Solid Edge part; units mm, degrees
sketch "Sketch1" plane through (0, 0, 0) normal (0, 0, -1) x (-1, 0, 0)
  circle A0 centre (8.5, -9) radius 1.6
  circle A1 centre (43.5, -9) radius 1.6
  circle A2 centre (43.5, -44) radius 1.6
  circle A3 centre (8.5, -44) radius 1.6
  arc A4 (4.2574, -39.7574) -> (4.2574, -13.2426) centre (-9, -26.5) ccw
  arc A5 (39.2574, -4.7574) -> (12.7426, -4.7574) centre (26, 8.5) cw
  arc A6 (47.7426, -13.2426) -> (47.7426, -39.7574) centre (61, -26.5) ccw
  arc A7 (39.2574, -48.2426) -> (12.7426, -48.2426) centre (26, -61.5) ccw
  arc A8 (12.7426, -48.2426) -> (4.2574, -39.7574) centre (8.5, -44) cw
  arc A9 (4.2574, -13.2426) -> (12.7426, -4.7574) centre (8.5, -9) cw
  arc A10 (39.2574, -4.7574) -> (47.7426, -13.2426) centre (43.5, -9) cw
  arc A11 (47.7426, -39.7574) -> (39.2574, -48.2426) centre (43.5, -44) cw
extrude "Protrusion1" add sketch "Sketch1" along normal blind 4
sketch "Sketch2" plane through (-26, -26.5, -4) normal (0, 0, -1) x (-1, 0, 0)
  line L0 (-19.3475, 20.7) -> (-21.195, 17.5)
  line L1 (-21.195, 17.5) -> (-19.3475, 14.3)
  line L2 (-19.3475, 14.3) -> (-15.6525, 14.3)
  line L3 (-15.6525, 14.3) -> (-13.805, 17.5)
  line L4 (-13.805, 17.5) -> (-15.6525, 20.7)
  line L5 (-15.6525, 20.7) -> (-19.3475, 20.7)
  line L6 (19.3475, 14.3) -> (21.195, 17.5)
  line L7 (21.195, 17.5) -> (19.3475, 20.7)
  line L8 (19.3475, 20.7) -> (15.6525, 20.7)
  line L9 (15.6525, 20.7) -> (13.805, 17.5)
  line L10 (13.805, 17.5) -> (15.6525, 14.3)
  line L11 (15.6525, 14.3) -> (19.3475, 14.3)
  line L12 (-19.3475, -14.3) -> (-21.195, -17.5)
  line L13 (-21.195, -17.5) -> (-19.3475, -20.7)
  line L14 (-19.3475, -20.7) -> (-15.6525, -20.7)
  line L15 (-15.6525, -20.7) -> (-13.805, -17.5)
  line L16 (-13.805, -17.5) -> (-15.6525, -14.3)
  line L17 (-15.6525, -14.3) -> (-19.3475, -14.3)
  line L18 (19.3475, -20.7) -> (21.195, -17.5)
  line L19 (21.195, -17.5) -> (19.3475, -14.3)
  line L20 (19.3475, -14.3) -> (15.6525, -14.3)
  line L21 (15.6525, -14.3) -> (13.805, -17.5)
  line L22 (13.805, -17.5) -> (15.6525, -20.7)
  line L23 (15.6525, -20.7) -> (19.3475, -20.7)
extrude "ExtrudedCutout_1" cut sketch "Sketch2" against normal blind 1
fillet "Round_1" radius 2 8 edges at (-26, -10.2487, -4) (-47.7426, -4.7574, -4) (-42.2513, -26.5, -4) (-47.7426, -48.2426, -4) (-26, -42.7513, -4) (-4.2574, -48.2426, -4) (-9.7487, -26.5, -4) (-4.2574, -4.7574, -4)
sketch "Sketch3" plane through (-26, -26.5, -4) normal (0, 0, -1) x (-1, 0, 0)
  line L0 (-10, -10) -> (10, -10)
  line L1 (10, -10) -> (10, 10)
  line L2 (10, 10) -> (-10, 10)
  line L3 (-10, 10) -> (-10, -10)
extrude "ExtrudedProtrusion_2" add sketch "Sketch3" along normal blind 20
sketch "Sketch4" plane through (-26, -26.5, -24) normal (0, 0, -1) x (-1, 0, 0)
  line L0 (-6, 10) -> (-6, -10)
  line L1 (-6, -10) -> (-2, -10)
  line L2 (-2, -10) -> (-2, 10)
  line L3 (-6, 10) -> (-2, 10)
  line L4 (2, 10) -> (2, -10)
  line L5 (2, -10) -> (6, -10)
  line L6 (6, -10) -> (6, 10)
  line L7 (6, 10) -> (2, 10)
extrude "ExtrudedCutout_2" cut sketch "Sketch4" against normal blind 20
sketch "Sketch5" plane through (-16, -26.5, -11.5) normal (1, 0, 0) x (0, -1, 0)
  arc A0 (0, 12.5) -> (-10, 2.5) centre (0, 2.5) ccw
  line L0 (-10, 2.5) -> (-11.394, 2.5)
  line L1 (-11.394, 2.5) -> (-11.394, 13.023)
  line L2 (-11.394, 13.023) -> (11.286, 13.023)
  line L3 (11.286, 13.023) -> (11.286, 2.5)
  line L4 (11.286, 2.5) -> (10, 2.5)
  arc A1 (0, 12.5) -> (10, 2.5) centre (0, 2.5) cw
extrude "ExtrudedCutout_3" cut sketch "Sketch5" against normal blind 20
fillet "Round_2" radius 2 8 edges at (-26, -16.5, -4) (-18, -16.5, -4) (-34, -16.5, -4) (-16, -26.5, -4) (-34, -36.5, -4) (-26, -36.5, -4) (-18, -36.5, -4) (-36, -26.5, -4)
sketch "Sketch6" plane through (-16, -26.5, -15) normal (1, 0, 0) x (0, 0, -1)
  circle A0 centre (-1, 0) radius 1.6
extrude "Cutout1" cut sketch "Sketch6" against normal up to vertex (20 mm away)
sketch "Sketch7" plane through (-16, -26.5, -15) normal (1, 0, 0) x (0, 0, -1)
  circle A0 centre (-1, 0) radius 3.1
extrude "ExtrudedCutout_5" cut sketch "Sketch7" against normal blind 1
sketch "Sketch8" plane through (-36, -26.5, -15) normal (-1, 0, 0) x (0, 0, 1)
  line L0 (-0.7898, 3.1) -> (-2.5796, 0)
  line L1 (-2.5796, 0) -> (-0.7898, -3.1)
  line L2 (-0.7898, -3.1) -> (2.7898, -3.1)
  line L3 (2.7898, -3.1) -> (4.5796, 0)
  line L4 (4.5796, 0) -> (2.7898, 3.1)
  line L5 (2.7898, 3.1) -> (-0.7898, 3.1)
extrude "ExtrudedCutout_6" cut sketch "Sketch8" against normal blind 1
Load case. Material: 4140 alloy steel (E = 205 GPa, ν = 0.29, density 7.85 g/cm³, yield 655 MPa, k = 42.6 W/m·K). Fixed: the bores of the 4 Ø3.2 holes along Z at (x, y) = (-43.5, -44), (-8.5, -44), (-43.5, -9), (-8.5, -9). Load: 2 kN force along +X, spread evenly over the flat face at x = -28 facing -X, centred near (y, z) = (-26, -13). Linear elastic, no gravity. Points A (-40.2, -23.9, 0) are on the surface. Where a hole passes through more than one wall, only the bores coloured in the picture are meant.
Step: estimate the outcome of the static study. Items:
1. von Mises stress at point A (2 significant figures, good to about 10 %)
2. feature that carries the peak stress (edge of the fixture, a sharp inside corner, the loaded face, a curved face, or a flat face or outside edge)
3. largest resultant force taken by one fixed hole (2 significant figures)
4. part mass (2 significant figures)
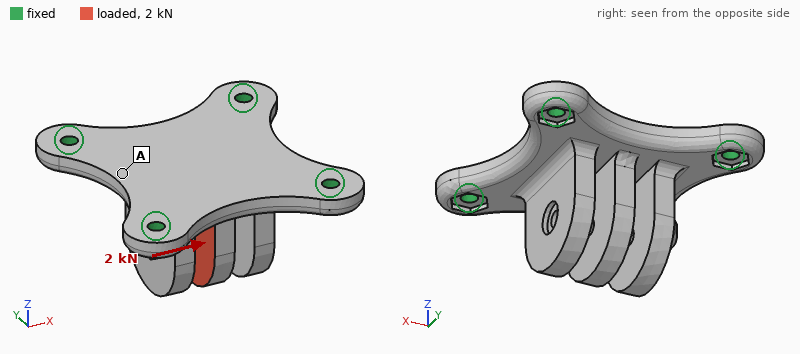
25 MPa
the loaded face
750 N
79 g
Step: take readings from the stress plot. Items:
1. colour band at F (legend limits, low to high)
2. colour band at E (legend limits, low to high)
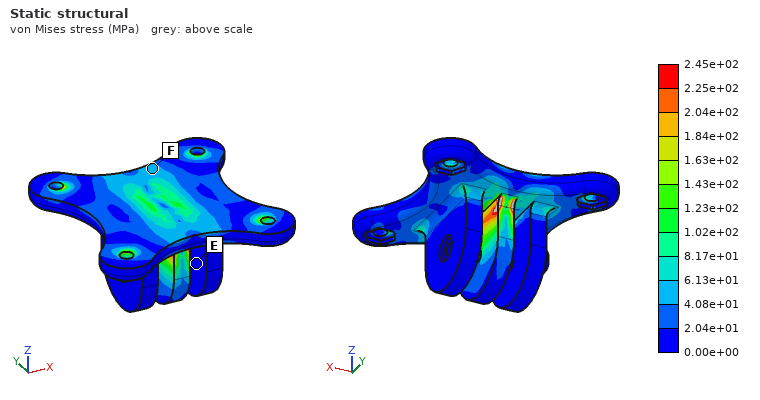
4.08e+01 to 6.13e+01 MPa
0.00e+00 to 2.04e+01 MPa
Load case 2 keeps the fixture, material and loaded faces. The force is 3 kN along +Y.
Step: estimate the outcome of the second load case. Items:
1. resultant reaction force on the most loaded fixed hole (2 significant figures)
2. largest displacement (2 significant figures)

1.1 kN
48 µm
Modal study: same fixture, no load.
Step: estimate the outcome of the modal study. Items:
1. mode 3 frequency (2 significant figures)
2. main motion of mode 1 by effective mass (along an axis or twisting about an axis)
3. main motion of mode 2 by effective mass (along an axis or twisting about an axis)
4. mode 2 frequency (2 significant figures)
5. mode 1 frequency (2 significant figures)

7900 Hz
along Z
along X
7400 Hz
6100 Hz
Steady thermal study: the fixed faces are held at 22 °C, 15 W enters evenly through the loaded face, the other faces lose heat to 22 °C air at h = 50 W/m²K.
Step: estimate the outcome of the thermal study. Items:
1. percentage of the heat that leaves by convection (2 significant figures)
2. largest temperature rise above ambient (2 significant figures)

32 %
67 K
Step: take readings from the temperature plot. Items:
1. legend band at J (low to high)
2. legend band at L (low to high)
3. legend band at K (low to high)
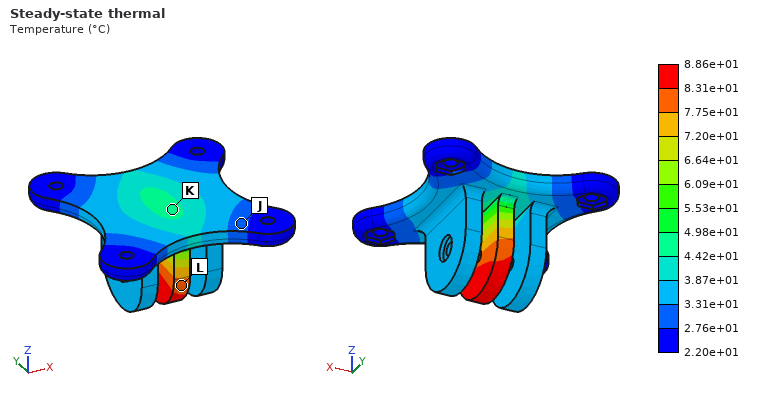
2.76e+01 to 3.31e+01 °C
7.75e+01 to 8.31e+01 °C
4.42e+01 to 4.98e+01 °C
